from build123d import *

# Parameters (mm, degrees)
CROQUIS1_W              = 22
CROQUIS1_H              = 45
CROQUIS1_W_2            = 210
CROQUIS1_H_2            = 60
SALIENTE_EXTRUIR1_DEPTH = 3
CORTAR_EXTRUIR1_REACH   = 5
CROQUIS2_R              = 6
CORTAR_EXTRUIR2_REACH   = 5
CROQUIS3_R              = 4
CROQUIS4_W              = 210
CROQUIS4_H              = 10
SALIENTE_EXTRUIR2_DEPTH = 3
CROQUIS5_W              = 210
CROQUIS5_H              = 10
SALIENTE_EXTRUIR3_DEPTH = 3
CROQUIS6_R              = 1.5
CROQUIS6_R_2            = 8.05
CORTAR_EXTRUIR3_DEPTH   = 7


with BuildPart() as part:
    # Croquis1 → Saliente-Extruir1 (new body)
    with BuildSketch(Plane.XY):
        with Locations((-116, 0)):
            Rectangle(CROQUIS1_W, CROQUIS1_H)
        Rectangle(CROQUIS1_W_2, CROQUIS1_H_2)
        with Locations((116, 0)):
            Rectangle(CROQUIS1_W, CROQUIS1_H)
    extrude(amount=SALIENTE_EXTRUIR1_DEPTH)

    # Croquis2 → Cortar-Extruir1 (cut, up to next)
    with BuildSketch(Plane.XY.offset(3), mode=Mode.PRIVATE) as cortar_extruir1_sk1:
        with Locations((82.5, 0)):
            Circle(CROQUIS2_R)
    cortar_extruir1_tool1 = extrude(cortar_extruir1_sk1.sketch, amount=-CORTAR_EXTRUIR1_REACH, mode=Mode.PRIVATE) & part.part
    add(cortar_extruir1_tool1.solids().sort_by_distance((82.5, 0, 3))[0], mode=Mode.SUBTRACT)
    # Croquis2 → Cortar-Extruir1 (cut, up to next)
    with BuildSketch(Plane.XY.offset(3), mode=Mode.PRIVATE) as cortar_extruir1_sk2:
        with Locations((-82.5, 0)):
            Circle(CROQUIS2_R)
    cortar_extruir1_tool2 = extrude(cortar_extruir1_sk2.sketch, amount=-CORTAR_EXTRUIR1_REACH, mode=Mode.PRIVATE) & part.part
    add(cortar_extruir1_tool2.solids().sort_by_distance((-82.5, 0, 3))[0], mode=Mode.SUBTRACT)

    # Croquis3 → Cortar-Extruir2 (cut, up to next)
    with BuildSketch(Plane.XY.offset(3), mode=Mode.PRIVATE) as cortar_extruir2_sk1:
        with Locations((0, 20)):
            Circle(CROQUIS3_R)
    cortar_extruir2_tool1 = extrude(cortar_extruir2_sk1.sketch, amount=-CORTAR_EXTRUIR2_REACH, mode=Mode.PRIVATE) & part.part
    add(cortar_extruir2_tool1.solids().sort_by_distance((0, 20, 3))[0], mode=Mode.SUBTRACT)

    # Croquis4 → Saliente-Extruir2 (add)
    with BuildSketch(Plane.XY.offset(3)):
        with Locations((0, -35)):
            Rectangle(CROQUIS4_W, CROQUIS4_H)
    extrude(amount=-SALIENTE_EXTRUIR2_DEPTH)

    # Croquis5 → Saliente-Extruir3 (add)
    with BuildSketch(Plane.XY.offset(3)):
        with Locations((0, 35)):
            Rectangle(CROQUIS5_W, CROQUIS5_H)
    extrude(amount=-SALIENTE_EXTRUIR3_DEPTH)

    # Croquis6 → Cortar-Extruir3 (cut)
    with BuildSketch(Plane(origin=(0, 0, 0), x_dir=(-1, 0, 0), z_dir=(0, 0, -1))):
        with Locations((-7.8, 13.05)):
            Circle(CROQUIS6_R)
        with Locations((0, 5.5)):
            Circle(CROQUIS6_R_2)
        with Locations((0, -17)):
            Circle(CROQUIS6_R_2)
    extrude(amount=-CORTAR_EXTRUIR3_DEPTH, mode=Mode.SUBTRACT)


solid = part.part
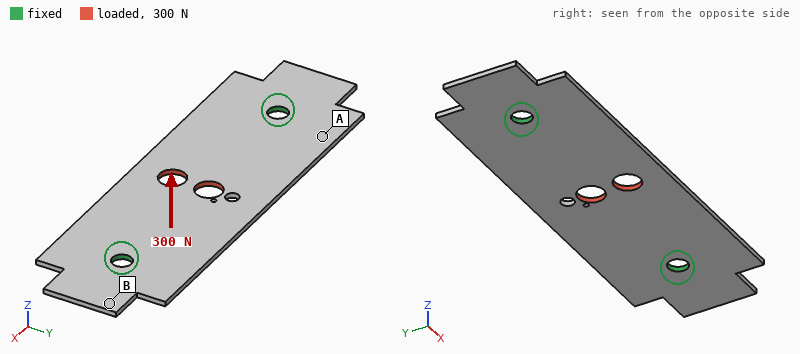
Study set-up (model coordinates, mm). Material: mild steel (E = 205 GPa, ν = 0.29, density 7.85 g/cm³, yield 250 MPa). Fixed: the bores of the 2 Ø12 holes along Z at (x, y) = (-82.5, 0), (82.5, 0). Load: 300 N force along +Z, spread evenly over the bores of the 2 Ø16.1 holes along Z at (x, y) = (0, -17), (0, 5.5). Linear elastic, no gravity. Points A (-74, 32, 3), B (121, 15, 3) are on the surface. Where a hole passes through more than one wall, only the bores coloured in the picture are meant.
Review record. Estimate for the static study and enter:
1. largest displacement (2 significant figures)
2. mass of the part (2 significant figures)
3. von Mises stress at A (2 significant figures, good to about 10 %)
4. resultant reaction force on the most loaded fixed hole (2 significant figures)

0.26 mm
430 g
22 MPa
150 N
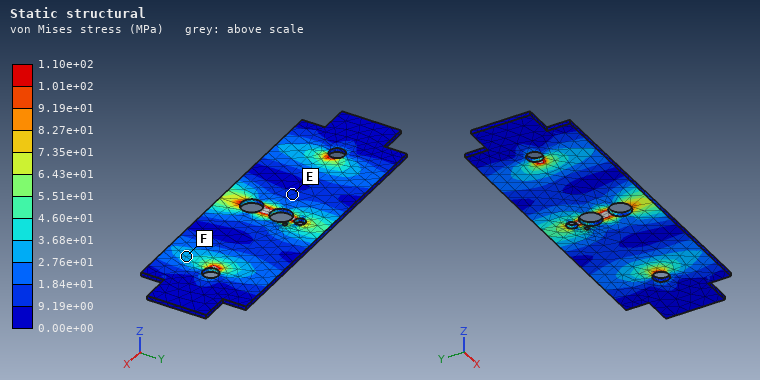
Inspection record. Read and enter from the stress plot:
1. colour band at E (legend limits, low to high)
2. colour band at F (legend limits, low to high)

9.19e+00 to 1.84e+01 MPa
2.76e+01 to 3.68e+01 MPa
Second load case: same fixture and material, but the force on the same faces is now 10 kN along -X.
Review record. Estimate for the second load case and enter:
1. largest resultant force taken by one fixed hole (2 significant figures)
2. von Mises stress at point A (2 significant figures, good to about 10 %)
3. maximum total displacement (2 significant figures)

5.0 kN
8.4 MPa
14 µm
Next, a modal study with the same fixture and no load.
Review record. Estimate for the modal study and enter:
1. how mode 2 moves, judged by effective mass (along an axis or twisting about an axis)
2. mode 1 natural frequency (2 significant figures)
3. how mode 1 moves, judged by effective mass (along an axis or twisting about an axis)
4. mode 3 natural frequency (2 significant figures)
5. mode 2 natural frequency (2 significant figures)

twisting about X
560 Hz
along Z
1400 Hz
760 Hz
